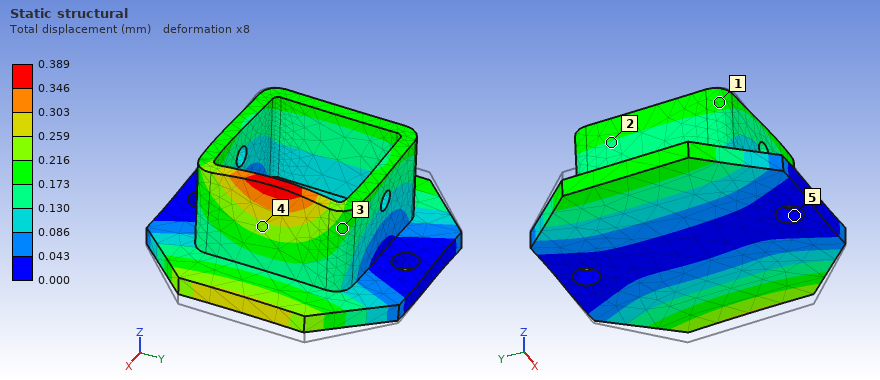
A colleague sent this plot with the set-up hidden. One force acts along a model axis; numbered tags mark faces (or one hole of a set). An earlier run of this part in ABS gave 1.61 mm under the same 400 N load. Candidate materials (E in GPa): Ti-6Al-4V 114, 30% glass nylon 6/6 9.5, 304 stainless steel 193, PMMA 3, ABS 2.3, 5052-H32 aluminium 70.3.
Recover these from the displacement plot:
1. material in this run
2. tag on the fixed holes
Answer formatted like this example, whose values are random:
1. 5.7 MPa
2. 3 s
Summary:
1. 30% glass nylon 6/6
2. 5
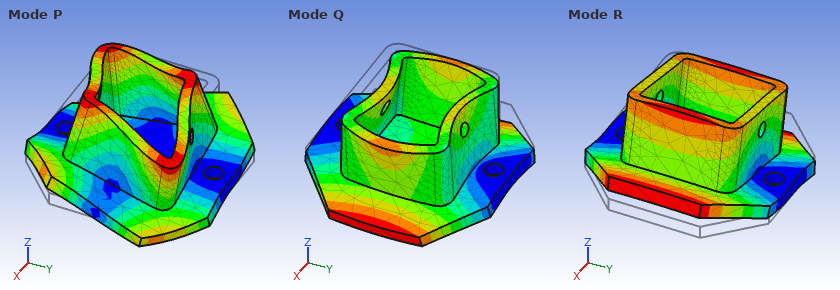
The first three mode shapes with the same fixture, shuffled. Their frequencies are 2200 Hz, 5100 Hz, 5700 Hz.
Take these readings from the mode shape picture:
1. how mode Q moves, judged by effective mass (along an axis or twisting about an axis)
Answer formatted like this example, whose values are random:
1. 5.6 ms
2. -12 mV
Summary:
1. along Z
